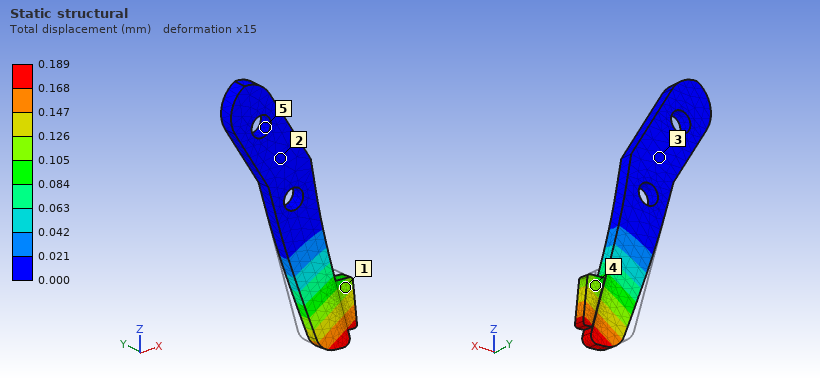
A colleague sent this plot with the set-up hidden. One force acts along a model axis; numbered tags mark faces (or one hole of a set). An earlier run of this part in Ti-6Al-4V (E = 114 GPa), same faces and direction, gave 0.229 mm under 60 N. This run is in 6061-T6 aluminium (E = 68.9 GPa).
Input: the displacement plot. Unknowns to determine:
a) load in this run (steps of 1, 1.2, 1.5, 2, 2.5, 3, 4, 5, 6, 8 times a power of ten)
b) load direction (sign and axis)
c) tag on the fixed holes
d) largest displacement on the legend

30 N
-Y
5
0.189 mm
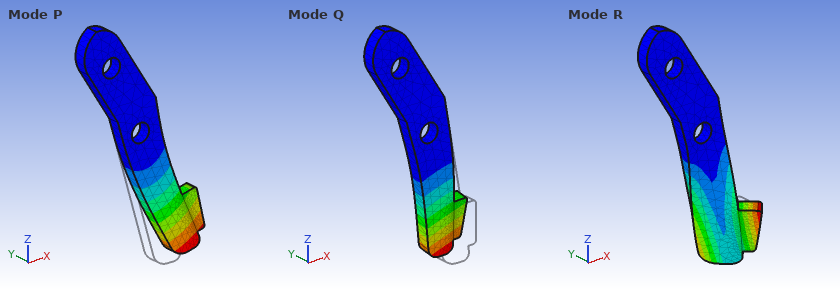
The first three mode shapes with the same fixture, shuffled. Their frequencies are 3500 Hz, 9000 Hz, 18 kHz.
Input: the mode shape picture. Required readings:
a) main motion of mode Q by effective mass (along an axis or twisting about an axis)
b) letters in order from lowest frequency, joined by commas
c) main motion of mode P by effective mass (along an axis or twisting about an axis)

along Y
Q, P, R
along X
